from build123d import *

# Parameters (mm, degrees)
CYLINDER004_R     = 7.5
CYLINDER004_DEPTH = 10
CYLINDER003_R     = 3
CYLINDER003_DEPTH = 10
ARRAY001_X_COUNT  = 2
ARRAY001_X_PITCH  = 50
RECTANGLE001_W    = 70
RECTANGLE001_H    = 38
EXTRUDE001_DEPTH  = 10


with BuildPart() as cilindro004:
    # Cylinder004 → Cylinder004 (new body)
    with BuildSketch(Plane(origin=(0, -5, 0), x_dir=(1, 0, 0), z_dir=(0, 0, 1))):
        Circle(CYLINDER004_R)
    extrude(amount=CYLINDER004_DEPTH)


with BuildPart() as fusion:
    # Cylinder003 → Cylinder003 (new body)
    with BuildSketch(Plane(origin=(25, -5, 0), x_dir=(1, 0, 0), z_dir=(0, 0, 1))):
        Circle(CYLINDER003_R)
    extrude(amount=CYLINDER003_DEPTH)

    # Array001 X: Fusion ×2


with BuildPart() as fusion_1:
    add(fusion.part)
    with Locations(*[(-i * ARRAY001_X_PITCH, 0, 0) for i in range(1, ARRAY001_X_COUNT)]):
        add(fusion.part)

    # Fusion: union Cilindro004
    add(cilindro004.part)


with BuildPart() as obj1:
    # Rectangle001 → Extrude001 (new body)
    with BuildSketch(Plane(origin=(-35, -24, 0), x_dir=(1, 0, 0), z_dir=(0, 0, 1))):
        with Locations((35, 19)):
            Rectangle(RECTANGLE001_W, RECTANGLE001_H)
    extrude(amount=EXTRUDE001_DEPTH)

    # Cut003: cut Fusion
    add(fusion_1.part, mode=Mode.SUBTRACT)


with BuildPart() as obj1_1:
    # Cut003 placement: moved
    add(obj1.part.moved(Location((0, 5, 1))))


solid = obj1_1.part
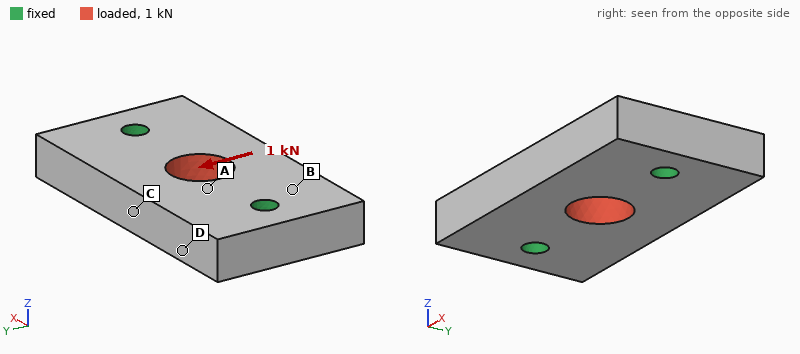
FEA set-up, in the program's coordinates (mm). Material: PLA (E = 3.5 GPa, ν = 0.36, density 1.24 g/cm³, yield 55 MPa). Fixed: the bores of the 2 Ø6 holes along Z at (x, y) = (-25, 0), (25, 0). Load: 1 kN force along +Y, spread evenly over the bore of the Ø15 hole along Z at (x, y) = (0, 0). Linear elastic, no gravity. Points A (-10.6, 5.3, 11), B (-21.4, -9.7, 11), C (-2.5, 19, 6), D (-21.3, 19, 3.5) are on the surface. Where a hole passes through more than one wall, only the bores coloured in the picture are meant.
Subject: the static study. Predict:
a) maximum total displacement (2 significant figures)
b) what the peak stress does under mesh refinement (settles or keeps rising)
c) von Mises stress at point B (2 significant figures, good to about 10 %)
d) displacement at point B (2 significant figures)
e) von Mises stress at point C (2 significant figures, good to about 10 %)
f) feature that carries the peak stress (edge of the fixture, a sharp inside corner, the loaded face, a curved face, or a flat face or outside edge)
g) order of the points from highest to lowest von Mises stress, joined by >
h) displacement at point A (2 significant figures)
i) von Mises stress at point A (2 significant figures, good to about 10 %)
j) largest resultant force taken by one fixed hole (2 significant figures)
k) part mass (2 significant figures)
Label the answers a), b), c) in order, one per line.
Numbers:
a) 40 µm
b) keeps rising
c) 1.9 MPa
d) 10 µm
e) 4.8 MPa
f) edge of the fixture
g) C > A > B > D
h) 27 µm
i) 3.0 MPa
j) 500 N
k) 30 g
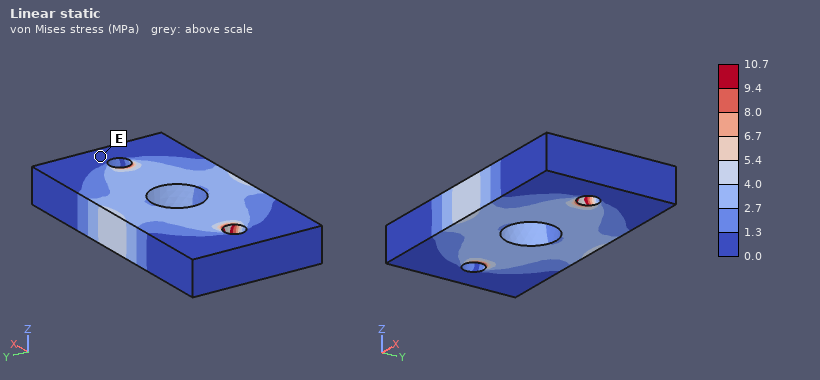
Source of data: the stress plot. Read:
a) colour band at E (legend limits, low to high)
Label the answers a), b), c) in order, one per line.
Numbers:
a) 0.0 to 1.3 MPa
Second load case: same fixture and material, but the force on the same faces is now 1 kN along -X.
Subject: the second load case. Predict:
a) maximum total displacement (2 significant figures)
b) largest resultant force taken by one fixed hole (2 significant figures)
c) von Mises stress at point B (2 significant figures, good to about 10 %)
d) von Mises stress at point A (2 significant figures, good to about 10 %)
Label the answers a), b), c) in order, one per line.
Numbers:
a) 17 µm
b) 500 N
c) 0.85 MPa
d) 2.7 MPa
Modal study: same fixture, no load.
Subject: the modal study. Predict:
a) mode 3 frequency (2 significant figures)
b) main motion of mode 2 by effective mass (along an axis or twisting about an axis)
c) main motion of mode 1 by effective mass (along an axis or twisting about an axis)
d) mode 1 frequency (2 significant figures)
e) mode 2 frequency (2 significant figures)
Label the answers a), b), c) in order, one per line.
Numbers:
a) 6500 Hz
b) along Z
c) twisting about X
d) 4100 Hz
e) 4500 Hz
